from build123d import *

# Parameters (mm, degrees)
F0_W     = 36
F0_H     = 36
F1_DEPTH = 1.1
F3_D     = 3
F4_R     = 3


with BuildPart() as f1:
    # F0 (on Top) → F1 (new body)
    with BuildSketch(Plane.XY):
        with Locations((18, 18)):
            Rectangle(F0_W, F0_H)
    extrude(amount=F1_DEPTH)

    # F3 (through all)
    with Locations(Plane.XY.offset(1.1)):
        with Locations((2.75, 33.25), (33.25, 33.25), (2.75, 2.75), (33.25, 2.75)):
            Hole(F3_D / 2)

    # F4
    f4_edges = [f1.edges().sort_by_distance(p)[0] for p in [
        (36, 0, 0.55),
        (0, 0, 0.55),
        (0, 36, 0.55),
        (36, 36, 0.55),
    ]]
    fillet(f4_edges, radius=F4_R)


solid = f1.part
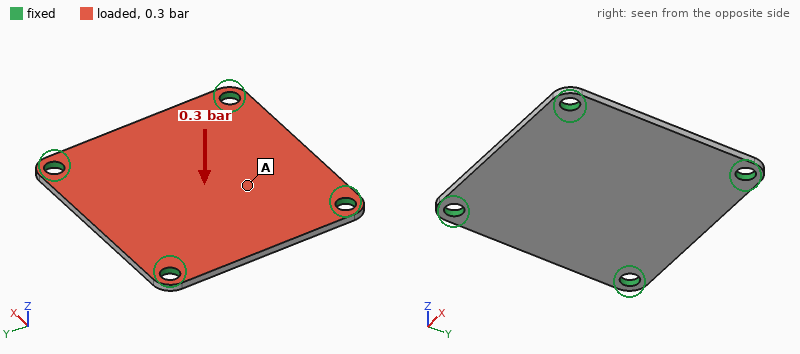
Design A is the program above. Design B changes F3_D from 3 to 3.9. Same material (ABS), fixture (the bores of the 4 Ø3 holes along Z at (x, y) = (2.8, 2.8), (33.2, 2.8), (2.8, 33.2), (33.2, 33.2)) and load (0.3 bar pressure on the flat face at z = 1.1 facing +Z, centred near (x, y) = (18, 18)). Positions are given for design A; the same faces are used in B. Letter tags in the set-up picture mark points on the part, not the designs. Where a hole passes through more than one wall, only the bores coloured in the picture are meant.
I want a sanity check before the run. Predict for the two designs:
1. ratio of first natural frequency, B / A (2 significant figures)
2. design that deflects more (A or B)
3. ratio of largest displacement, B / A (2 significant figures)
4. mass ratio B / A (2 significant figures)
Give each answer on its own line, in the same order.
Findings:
1.1
A
0.88
0.98
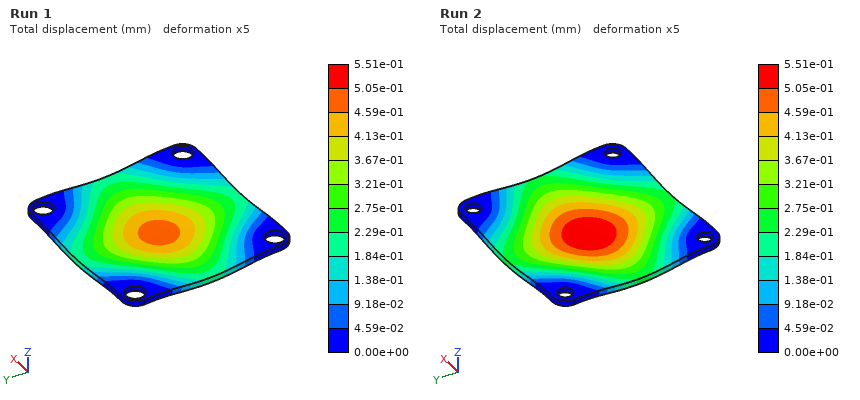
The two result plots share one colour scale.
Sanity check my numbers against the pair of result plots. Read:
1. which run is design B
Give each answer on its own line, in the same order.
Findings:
Run 1
